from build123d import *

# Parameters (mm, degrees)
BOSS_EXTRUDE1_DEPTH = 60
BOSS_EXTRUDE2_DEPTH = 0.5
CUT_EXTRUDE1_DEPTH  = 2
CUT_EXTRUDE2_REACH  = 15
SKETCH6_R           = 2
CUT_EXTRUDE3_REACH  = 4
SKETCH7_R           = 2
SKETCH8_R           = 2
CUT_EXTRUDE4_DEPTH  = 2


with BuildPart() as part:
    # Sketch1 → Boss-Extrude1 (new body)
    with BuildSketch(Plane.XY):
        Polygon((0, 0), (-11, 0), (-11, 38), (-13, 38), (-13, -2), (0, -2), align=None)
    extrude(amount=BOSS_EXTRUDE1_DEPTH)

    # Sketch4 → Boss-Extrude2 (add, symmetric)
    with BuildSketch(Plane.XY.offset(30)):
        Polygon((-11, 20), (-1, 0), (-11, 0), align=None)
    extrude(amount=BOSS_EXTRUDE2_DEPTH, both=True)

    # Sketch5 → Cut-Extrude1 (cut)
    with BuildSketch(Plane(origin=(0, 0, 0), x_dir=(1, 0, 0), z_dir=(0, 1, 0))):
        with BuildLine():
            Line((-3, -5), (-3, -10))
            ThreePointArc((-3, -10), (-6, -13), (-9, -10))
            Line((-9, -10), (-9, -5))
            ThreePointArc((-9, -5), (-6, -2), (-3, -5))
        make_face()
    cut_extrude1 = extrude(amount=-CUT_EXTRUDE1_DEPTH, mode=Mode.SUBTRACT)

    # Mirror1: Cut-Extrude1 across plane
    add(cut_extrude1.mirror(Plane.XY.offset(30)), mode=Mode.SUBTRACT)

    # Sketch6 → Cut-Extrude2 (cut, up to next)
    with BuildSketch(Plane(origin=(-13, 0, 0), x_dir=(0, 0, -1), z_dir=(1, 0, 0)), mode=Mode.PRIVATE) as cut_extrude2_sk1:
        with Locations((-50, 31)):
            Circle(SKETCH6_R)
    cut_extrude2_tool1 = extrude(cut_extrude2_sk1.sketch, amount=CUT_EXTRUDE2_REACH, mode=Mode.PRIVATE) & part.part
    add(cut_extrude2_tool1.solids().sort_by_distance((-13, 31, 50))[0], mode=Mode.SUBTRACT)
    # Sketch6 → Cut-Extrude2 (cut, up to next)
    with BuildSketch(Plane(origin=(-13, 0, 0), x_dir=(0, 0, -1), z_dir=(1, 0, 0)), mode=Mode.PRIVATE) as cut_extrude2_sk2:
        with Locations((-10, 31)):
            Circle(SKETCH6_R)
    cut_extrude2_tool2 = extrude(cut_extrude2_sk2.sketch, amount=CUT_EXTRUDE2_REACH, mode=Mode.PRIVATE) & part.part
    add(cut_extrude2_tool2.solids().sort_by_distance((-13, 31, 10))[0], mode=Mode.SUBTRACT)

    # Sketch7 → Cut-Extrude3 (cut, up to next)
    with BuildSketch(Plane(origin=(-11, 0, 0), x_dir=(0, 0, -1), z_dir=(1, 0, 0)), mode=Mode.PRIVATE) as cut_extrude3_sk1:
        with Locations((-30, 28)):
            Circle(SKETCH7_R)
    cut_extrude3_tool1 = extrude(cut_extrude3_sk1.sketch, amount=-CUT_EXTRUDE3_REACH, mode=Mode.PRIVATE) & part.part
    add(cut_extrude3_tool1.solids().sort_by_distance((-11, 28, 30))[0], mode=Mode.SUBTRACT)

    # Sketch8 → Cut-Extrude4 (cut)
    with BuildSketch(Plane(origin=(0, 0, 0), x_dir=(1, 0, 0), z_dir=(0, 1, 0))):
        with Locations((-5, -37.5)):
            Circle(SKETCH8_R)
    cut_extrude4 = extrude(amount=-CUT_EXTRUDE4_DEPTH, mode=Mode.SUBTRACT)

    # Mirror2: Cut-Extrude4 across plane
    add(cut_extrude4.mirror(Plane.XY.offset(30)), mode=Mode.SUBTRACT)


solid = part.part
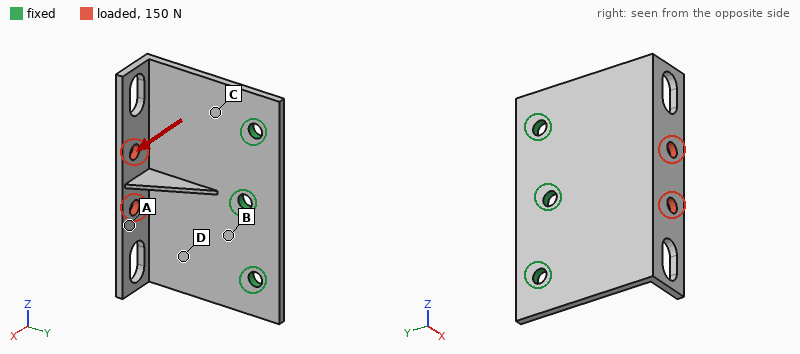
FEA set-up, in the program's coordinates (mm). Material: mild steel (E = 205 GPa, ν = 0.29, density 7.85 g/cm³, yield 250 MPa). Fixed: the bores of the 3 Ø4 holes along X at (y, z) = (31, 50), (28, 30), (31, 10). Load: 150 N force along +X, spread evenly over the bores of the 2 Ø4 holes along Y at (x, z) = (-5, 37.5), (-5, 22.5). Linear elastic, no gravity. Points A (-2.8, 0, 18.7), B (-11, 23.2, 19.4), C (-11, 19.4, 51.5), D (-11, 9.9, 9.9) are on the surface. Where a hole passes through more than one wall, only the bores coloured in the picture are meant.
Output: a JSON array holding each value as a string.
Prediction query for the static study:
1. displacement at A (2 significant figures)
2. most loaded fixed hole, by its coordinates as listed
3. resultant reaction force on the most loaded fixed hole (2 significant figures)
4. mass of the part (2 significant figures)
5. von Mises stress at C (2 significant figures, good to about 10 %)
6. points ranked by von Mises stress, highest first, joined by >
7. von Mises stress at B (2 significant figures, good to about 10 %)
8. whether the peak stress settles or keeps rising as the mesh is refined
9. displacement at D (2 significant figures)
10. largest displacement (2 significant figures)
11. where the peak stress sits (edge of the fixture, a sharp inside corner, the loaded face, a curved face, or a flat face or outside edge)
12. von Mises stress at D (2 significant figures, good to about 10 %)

["0.16 mm", "(28, 30)", "110 N", "46 g", "59 MPa", "B > C > D > A", "79 MPa", "keeps rising", "0.077 mm", "0.18 mm", "edge of the fixture", "30 MPa"]
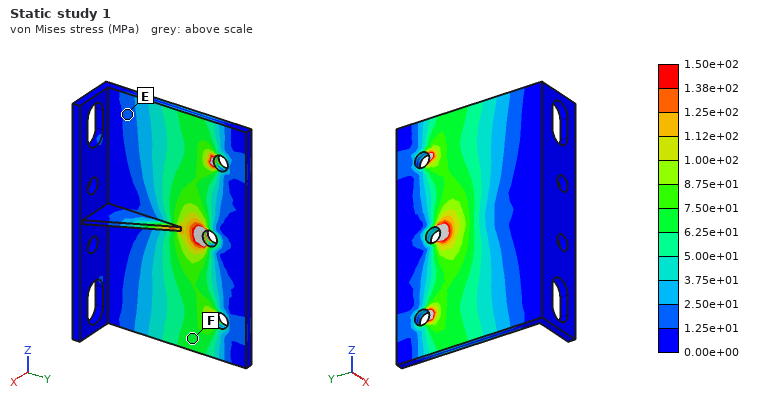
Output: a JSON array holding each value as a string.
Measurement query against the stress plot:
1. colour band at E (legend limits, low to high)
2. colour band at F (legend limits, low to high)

["1.25e+01 to 2.50e+01 MPa", "6.25e+01 to 7.50e+01 MPa"]
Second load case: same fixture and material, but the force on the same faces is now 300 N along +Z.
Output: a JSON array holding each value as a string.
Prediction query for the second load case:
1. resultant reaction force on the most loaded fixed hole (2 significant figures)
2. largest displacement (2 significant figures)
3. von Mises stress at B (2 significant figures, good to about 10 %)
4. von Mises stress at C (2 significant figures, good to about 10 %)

["230 N", "84 µm", "26 MPa", "25 MPa"]
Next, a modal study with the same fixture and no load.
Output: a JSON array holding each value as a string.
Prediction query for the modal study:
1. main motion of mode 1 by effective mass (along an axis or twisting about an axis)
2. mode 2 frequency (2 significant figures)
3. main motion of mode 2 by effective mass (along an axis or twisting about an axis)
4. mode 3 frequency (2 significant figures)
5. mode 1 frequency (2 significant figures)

["along X", "2000 Hz", "twisting about Y", "6600 Hz", "1200 Hz"]
